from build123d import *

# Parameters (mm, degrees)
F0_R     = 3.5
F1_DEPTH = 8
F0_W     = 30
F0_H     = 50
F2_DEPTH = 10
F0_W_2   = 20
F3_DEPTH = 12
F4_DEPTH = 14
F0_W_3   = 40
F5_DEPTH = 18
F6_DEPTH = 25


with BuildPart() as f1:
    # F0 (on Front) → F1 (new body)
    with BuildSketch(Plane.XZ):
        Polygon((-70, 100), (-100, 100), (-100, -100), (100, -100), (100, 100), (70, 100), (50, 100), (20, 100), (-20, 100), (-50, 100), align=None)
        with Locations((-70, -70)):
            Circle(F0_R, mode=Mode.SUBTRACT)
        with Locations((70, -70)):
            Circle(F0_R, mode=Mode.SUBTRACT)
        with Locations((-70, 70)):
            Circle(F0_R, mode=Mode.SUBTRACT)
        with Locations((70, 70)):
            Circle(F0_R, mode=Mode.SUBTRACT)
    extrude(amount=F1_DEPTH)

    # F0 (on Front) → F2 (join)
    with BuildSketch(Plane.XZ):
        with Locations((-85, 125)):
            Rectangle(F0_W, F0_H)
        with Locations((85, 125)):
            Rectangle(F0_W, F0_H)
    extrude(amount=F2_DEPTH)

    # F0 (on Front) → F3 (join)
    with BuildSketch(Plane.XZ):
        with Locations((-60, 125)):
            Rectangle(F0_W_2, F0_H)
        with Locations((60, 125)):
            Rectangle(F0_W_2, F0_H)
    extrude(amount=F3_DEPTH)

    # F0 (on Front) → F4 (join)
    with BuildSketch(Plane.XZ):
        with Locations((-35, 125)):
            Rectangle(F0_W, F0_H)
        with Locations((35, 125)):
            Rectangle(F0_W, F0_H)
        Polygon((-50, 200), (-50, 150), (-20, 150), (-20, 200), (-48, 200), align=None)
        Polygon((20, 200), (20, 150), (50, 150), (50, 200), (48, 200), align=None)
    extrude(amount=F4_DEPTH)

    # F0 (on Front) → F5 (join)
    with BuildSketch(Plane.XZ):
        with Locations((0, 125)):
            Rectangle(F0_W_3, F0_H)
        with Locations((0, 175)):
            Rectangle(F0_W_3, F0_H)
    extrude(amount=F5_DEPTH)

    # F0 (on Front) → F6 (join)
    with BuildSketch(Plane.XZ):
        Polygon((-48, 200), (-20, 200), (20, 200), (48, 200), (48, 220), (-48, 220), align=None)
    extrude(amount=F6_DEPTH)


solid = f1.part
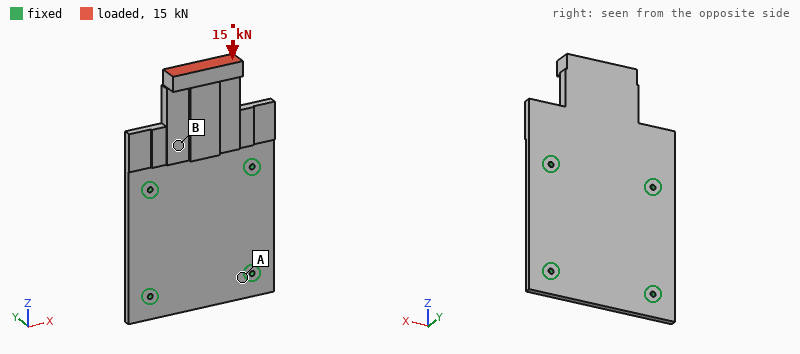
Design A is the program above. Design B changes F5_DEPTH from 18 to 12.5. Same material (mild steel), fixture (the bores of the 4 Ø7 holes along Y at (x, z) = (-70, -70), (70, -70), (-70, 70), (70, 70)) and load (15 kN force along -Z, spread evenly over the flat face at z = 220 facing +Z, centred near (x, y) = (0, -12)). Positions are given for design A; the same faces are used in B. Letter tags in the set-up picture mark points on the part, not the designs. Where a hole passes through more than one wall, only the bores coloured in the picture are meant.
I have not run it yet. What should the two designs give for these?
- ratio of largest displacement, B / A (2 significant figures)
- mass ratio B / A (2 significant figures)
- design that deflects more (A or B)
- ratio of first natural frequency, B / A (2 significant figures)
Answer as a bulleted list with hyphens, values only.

- 1.1
- 0.96
- B
- 1.0
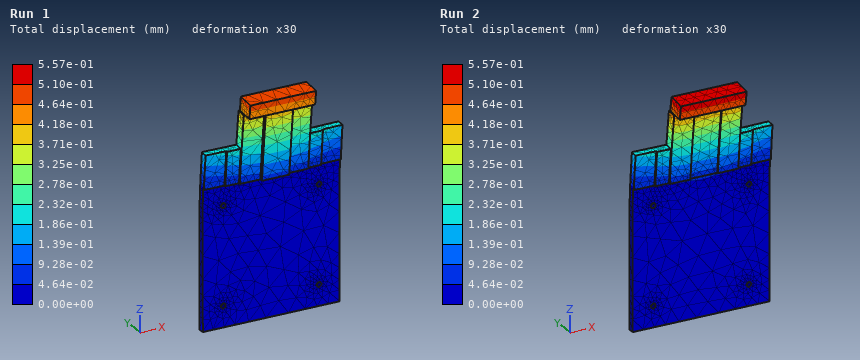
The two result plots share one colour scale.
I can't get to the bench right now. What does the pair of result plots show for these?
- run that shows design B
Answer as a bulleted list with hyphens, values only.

- Run 2
